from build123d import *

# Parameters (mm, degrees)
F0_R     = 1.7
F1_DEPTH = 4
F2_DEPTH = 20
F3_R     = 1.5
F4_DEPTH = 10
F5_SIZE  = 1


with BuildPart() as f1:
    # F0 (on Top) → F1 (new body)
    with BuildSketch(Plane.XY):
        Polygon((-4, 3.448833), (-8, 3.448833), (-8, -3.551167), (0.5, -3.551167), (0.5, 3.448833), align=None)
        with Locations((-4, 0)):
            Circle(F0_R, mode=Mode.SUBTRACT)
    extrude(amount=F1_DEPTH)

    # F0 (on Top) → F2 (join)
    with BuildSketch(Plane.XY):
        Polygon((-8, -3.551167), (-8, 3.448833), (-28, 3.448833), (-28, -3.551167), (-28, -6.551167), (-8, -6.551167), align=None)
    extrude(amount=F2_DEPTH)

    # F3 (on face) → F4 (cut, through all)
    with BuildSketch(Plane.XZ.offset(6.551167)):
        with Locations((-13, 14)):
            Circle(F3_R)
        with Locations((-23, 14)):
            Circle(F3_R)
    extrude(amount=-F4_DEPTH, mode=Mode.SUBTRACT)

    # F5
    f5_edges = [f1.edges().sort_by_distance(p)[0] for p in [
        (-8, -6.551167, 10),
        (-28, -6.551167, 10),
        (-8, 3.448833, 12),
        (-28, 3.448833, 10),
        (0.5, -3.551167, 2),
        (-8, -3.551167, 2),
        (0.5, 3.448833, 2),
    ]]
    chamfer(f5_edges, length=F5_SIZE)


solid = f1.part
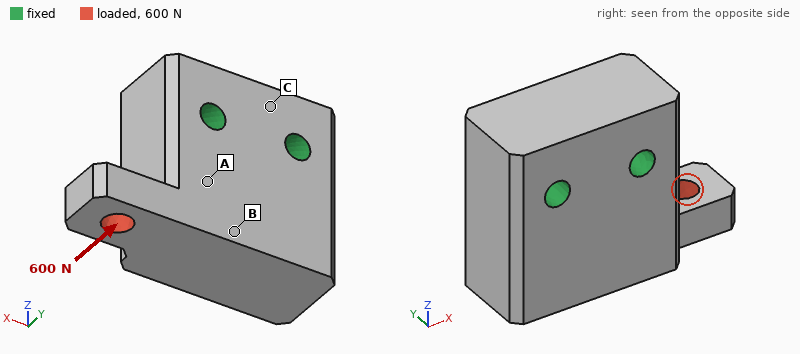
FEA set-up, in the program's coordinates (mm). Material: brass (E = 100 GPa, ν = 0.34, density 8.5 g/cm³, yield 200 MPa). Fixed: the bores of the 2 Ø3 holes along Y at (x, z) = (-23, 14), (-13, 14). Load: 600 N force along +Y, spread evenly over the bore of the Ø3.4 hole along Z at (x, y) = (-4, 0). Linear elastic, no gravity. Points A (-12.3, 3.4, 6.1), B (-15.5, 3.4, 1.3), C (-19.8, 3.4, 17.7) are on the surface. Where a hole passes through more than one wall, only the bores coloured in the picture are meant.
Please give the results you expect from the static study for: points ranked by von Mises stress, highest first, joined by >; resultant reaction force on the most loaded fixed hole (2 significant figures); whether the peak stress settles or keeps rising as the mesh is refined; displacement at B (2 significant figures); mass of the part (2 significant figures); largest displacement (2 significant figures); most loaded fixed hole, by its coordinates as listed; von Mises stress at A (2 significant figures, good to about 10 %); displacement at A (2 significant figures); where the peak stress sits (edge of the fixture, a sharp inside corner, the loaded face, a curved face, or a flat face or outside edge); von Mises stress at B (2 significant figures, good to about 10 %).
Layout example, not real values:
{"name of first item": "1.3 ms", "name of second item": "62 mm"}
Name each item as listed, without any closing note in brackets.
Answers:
{"points ranked by von Mises stress, highest first, joined by >": "A > B > C", "resultant reaction force on the most loaded fixed hole": "750 N", "whether the peak stress settles or keeps rising as the mesh is refined": "keeps rising", "displacement at B": "4.6 µm", "mass of the part": "34 g", "largest displacement": "29 µm", "most loaded fixed hole, by its coordinates as listed": "(-13, 14)", "von Mises stress at A": "39 MPa", "displacement at A": "4.5 µm", "where the peak stress sits": "a sharp inside corner", "von Mises stress at B": "27 MPa"}
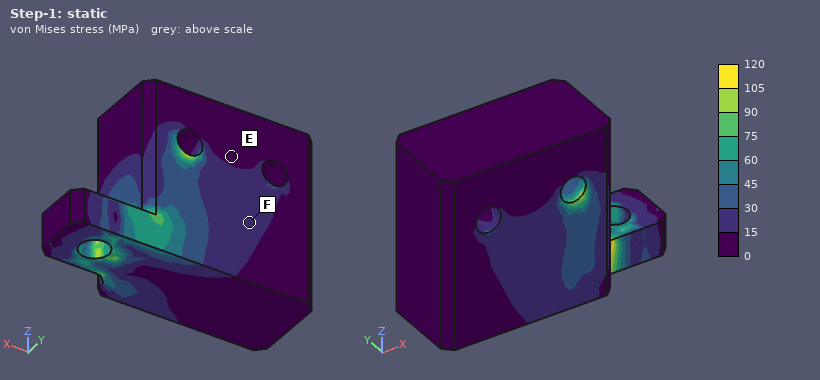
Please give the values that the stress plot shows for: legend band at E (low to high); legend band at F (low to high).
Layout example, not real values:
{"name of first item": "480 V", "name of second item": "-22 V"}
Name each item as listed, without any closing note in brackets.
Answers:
{"legend band at E": "0 to 15 MPa", "legend band at F": "15 to 30 MPa"}
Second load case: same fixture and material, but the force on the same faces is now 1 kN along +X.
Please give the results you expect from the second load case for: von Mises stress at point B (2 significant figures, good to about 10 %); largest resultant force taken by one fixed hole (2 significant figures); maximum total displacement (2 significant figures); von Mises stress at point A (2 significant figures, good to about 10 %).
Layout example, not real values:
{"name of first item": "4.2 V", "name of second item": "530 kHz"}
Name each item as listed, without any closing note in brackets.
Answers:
{"von Mises stress at point B": "24 MPa", "largest resultant force taken by one fixed hole": "1.1 kN", "maximum total displacement": "12 µm", "von Mises stress at point A": "20 MPa"}
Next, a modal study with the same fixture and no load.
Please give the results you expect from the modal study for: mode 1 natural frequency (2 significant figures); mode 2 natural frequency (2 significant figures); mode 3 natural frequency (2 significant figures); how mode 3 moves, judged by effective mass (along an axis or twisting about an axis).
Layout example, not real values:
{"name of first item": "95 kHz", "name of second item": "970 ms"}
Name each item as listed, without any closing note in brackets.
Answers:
{"mode 1 natural frequency": "17 kHz", "mode 2 natural frequency": "17 kHz", "mode 3 natural frequency": "23 kHz", "how mode 3 moves, judged by effective mass": "along Y"}
